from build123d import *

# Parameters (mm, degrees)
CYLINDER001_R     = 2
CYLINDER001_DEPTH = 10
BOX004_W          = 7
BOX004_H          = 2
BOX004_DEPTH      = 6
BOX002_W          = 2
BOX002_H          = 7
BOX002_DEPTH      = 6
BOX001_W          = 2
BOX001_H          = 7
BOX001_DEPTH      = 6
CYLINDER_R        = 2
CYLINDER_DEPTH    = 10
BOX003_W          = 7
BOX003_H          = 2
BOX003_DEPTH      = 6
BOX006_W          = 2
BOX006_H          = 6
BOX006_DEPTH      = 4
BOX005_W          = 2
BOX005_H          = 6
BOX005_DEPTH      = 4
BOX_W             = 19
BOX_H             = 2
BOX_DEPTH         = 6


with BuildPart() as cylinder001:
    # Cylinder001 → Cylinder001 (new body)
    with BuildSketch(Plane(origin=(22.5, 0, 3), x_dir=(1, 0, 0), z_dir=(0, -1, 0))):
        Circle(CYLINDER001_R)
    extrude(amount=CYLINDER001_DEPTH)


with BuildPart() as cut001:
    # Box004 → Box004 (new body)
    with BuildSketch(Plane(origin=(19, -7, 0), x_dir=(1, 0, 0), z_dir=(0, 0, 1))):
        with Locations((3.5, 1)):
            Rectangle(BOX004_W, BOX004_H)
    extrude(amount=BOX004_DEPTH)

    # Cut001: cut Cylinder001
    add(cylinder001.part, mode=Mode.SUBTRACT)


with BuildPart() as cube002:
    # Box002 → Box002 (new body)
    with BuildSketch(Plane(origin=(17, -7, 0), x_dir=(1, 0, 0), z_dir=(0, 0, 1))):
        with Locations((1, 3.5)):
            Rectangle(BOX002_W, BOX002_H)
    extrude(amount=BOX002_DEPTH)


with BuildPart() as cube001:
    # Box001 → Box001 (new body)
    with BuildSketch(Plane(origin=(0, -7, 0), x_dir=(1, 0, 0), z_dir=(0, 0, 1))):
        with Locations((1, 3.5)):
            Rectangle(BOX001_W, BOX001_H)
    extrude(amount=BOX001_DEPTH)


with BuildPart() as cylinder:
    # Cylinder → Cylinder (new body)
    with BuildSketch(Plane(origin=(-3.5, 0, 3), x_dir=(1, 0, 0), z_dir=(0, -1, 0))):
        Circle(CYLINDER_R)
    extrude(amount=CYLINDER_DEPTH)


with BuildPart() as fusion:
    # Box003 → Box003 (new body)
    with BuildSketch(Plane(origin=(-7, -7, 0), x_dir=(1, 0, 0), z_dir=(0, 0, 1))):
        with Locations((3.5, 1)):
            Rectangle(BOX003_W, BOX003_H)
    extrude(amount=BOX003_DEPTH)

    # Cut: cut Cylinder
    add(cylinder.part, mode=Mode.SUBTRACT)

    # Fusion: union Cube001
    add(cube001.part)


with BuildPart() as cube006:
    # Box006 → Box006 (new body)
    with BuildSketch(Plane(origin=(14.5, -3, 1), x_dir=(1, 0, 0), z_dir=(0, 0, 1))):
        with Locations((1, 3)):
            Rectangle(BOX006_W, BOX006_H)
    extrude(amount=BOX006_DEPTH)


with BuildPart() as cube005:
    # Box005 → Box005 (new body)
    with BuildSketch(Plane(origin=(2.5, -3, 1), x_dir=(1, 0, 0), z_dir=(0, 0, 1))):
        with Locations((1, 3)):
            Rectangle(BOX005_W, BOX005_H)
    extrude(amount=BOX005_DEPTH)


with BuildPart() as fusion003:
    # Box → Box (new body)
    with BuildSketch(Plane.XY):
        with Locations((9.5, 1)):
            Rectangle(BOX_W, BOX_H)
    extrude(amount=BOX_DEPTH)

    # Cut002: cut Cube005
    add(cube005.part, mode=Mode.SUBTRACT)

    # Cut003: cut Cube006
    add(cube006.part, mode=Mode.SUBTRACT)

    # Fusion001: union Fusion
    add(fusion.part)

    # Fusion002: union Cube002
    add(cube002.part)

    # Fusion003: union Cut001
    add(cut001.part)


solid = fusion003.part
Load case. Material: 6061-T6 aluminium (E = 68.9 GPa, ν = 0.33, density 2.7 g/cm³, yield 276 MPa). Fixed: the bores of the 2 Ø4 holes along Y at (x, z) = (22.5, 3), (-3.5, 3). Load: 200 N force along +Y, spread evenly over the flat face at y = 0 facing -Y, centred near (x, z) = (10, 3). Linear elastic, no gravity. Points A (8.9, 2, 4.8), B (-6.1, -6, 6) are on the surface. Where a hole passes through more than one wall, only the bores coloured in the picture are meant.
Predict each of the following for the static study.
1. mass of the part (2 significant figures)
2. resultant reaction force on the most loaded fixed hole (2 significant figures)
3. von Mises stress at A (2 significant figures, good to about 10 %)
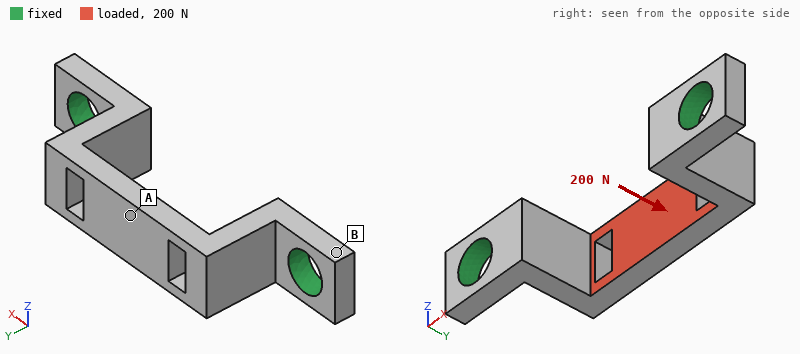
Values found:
1.3 g
120 N
67 MPa
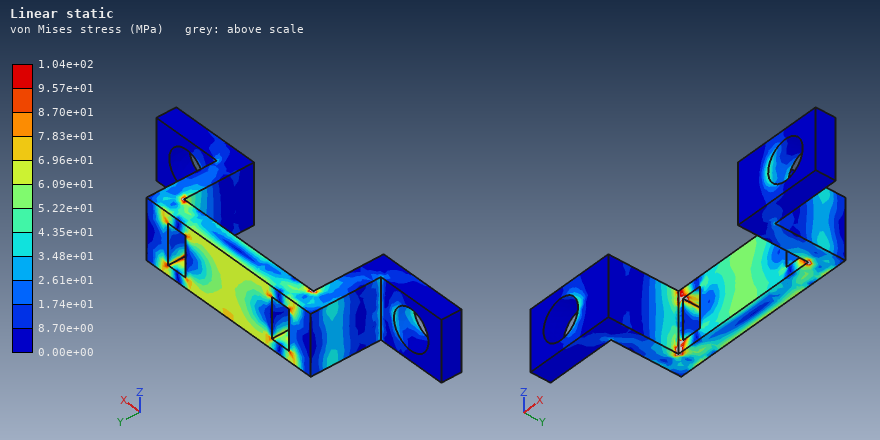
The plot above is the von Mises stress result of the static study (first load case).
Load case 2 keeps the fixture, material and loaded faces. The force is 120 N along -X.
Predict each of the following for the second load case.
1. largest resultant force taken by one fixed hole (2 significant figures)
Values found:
61 N
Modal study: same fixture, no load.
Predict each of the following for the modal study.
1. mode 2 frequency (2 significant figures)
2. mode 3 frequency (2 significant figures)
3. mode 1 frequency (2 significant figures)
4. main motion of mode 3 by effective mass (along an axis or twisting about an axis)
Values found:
14 kHz
23 kHz
14 kHz
along Y
